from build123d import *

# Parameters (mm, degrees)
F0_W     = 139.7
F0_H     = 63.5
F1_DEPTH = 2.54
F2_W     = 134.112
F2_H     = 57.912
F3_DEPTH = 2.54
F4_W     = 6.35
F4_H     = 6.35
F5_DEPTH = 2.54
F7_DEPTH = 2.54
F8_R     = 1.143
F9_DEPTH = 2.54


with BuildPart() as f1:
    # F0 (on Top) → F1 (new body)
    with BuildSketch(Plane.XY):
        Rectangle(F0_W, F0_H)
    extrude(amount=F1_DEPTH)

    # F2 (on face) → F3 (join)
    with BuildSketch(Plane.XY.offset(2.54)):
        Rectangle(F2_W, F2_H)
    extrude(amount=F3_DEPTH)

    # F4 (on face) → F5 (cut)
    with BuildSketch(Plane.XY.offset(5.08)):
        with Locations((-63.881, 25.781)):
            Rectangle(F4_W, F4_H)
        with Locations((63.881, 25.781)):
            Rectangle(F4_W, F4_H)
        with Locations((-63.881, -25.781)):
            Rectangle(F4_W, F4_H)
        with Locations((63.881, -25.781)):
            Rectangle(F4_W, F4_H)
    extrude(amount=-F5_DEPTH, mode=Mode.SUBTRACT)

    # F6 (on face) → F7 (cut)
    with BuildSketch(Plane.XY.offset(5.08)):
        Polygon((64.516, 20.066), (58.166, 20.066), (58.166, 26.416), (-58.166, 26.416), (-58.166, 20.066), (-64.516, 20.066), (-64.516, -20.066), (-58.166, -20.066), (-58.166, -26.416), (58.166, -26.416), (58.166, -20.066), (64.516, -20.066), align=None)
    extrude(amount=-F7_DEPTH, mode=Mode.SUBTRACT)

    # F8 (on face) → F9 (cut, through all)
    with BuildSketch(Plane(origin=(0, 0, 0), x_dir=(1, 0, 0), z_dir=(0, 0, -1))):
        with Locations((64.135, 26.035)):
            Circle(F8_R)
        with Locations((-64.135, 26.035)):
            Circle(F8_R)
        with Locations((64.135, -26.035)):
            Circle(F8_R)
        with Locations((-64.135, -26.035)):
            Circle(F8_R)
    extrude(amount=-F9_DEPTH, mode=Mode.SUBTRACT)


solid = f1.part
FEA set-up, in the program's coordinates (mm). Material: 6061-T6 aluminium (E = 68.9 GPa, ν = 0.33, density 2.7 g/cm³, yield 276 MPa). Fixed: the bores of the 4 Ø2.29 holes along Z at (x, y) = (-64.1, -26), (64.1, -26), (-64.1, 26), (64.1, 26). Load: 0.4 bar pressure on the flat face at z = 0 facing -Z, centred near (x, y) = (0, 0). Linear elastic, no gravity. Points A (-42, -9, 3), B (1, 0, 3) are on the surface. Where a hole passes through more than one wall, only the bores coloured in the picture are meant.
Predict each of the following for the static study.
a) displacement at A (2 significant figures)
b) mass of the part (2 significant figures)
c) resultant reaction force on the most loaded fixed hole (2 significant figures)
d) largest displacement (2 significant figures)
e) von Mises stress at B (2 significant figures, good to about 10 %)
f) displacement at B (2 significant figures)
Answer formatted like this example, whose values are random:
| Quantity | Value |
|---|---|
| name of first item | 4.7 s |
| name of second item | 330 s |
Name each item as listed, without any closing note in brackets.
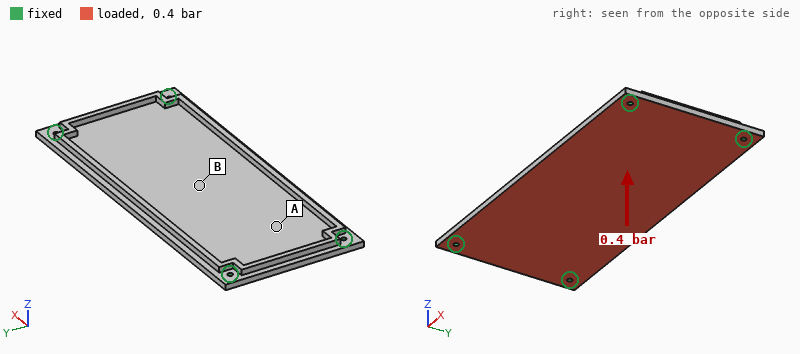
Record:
| Quantity | Value |
|---|---|
| displacement at A | 0.11 mm |
| mass of the part | 67 g |
| resultant reaction force on the most loaded fixed hole | 95 N |
| largest displacement | 0.25 mm |
| von Mises stress at B | 16 MPa |
| displacement at B | 0.25 mm |
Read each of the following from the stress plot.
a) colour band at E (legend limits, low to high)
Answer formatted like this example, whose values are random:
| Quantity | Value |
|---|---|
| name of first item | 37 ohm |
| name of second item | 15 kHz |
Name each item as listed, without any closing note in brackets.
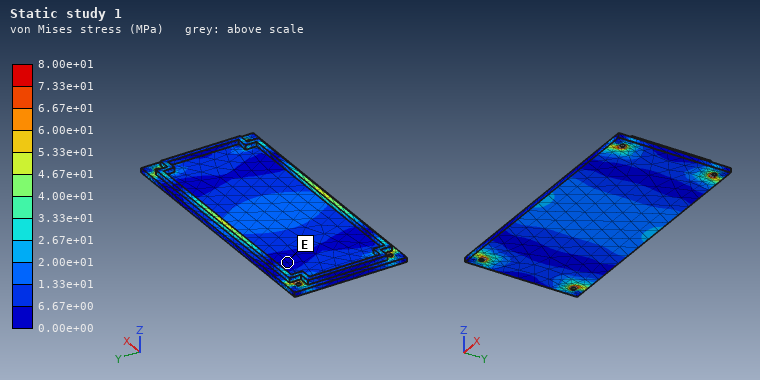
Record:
| Quantity | Value |
|---|---|
| colour band at E | 0.00e+00 to 6.67e+00 MPa |
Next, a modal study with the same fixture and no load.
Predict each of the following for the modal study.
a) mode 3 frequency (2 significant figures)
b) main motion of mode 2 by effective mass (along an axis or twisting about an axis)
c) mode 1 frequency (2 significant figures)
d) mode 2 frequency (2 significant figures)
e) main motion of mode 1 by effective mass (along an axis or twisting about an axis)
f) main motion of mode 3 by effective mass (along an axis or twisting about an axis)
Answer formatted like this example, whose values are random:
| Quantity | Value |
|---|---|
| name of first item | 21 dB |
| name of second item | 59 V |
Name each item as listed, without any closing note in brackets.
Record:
| Quantity | Value |
|---|---|
| mode 3 frequency | 2400 Hz |
| main motion of mode 2 by effective mass | twisting about X |
| mode 1 frequency | 850 Hz |
| mode 2 frequency | 1500 Hz |
| main motion of mode 1 by effective mass | along Z |
| main motion of mode 3 by effective mass | twisting about Y |
